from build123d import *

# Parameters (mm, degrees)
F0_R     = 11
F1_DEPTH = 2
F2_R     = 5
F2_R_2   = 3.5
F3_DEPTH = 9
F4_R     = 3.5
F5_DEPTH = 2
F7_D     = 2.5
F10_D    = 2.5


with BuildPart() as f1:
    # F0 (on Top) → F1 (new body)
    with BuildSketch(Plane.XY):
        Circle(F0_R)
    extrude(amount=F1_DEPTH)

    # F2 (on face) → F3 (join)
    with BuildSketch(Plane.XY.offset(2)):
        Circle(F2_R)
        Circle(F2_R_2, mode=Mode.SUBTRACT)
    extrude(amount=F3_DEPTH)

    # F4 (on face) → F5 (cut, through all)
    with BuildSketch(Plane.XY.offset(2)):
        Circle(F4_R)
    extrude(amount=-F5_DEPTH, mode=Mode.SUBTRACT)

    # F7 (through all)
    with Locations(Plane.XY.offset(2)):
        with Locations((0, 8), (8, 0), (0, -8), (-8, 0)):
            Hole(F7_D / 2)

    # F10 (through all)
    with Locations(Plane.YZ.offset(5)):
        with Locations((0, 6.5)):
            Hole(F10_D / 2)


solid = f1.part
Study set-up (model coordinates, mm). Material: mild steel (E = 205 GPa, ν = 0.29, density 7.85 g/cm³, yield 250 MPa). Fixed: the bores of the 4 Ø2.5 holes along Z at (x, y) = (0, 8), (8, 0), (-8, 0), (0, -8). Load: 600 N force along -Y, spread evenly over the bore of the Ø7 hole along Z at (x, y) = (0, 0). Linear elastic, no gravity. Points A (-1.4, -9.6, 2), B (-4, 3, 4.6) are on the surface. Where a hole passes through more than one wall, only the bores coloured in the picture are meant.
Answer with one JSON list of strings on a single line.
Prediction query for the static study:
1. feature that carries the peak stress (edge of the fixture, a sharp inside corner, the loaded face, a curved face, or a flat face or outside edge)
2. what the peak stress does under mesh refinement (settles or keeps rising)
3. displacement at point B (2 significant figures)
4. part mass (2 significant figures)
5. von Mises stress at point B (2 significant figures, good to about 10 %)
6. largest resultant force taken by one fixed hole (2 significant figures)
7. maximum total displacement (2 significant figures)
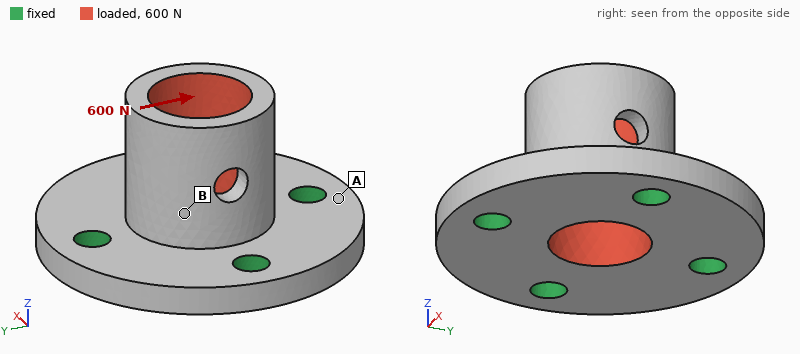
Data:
["edge of the fixture", "keeps rising", "1.9 µm", "7.8 g", "17 MPa", "270 N", "5.2 µm"]
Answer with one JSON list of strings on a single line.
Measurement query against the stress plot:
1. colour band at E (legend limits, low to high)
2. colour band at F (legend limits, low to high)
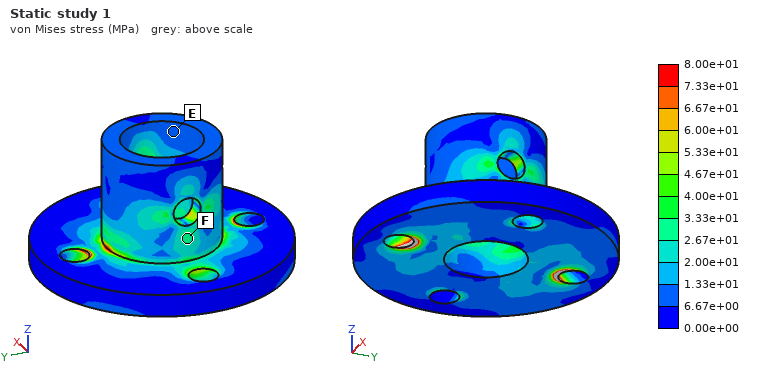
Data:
["6.67e+00 to 1.33e+01 MPa", "2.67e+01 to 3.33e+01 MPa"]
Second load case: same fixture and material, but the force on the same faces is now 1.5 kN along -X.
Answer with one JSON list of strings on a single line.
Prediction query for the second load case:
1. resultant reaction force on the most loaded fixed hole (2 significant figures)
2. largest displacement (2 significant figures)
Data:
["680 N", "12 µm"]
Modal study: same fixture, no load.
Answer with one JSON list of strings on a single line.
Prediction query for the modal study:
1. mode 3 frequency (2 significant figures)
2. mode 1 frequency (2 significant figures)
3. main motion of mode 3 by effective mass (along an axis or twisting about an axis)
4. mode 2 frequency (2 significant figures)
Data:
["55 kHz", "34 kHz", "along Z", "35 kHz"]
